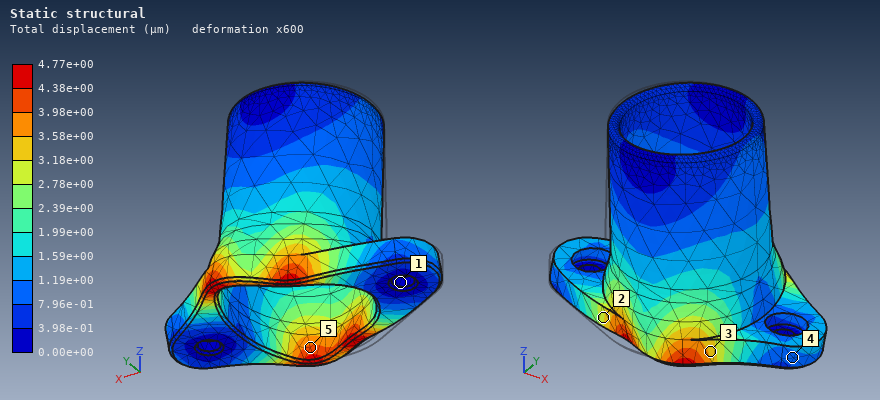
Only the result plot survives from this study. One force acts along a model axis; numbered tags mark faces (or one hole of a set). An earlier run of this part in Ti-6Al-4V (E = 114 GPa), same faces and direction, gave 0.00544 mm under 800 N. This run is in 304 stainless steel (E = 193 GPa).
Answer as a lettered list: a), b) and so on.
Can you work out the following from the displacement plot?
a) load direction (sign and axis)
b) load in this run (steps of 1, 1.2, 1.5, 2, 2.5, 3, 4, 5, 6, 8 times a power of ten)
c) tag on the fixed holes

a) +X
b) 1.2 kN
c) 1
